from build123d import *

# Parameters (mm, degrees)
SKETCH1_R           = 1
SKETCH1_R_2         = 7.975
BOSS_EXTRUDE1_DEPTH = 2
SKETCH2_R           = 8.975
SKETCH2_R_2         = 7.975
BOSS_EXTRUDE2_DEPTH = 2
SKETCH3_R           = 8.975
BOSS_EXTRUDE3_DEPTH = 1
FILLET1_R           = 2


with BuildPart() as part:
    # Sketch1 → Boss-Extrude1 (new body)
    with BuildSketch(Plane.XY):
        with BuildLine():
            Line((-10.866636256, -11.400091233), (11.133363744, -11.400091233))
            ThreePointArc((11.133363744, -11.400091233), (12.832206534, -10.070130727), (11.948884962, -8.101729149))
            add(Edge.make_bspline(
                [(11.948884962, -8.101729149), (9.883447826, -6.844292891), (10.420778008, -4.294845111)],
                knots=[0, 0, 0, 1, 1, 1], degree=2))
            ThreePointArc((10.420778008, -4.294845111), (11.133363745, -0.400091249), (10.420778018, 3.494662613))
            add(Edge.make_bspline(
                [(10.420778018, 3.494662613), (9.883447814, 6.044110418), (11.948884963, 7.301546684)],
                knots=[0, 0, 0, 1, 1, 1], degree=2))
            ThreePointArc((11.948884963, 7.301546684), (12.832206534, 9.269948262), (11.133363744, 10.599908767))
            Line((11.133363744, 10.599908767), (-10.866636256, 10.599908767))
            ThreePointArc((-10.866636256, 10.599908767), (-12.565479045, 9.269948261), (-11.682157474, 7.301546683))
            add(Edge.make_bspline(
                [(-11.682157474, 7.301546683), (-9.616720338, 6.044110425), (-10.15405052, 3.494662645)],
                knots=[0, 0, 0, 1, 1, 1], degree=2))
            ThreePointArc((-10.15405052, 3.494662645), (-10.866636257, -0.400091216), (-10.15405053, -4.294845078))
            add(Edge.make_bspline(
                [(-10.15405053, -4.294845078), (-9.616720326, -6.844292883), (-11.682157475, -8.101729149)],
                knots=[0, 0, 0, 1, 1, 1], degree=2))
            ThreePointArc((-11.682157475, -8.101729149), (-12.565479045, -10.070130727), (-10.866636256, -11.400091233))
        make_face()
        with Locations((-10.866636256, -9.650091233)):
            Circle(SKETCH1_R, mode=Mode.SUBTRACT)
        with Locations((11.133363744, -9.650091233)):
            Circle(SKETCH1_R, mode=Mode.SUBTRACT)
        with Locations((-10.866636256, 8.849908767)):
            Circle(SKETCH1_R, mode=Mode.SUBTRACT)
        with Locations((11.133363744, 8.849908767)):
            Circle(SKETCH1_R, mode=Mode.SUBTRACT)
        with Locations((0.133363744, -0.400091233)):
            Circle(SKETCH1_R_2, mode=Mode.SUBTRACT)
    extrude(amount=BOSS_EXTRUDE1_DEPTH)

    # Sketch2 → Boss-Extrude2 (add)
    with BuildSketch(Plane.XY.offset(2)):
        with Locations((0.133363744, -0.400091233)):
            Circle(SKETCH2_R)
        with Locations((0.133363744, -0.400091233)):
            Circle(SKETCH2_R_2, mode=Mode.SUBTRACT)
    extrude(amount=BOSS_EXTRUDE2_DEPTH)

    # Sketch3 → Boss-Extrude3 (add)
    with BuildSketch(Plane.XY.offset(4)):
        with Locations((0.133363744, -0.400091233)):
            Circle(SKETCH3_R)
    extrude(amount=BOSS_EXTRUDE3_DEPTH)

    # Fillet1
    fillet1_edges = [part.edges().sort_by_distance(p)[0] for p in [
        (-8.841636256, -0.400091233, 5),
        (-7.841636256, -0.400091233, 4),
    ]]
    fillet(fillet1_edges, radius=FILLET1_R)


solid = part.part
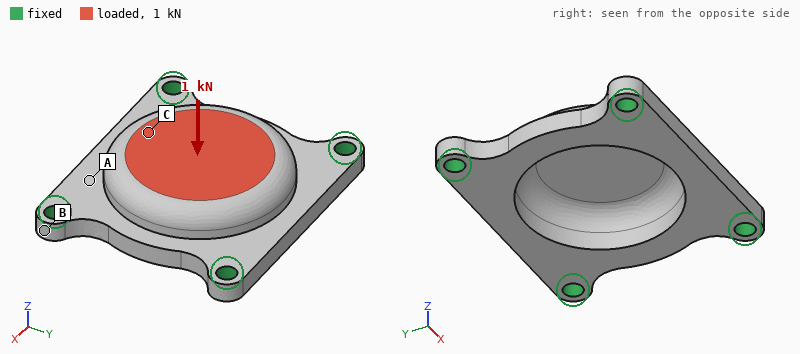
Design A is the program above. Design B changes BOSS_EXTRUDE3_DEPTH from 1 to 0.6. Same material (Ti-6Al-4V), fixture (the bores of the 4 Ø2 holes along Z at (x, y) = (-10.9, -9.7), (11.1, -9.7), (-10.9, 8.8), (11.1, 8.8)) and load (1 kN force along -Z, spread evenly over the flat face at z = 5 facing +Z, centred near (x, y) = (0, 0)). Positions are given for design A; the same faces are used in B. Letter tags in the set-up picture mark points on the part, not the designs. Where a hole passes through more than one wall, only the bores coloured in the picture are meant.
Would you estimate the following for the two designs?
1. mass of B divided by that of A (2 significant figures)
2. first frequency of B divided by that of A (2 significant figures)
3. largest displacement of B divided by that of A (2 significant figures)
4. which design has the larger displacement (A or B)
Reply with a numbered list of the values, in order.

1. 0.89
2. 1.0
3. 2.7
4. B
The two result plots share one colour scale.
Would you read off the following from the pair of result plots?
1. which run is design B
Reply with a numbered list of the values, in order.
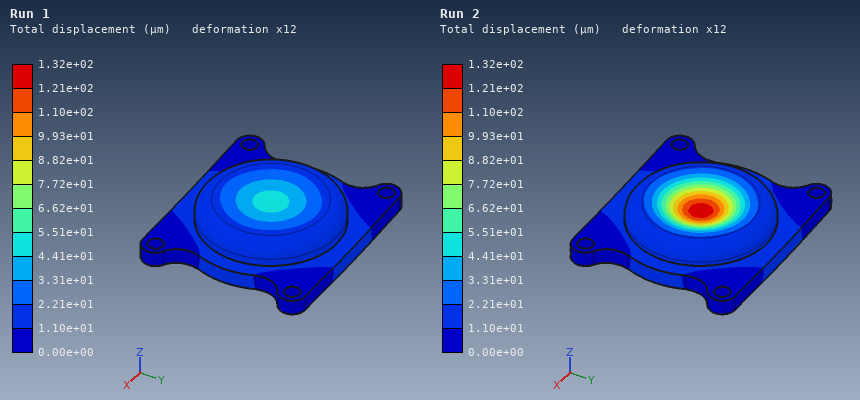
1. Run 2
